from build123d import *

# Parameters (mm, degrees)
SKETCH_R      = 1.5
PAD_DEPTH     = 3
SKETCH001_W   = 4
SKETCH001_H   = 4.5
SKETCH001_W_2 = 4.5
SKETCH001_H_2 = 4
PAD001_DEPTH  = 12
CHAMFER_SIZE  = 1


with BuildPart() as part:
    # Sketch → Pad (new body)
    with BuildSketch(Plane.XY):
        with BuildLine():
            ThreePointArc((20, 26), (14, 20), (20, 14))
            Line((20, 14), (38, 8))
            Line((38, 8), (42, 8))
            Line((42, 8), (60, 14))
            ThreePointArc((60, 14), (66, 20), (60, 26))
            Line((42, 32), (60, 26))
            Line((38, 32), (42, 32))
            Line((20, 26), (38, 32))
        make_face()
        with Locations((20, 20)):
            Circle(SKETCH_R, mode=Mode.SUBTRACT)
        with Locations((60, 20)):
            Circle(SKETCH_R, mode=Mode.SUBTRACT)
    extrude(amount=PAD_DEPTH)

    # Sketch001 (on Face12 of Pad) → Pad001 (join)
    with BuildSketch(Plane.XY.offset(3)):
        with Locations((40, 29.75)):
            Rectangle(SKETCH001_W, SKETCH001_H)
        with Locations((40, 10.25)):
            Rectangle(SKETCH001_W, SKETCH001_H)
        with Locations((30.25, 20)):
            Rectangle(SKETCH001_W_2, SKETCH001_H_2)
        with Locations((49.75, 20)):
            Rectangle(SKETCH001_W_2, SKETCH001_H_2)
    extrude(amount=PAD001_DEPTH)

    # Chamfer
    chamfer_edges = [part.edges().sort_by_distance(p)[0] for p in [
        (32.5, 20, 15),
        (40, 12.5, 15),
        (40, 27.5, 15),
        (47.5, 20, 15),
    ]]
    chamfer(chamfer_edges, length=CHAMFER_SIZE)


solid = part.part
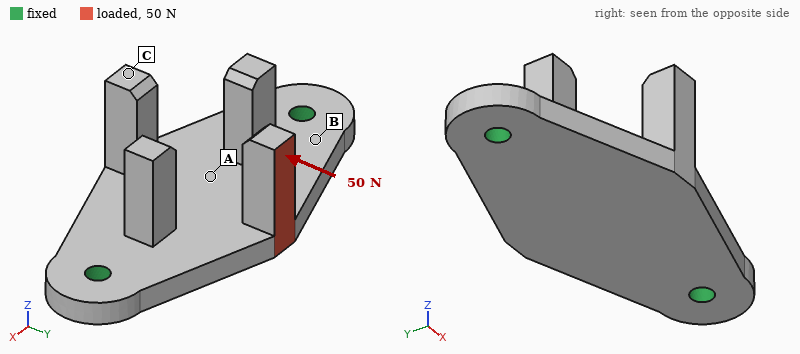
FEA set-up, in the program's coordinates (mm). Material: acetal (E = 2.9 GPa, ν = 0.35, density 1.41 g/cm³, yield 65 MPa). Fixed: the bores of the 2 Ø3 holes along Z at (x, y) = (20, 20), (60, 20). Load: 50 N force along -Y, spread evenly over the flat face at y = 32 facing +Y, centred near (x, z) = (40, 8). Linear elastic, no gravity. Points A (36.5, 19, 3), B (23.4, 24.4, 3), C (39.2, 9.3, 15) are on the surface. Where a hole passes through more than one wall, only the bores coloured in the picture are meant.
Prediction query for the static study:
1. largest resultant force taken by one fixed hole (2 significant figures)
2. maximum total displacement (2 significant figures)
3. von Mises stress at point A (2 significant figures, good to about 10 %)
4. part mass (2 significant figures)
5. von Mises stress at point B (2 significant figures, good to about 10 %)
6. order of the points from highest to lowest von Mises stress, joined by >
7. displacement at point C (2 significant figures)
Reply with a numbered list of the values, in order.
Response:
1. 25 N
2. 0.65 mm
3. 3.4 MPa
4. 4.8 g
5. 6.8 MPa
6. B > A > C
7. 0.19 mm
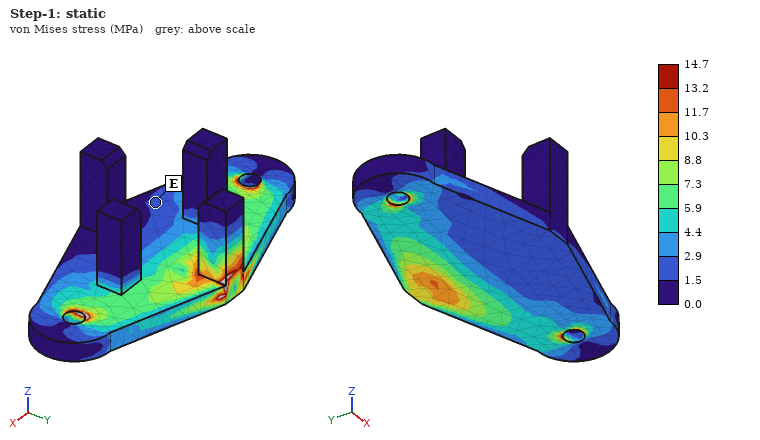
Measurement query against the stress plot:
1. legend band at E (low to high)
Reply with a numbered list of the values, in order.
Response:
1. 1.5 to 2.9 MPa
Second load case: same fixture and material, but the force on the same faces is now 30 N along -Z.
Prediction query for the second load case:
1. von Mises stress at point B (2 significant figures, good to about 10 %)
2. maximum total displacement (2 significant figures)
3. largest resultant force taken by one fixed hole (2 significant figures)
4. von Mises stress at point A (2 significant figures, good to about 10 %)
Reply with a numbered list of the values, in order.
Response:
1. 8.0 MPa
2. 0.54 mm
3. 15 N
4. 4.0 MPa
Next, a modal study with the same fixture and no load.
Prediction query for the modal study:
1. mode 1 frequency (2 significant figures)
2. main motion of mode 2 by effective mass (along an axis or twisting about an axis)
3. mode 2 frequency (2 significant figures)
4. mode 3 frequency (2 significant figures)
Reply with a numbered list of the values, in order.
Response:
1. 1600 Hz
2. along Z
3. 1800 Hz
4. 3300 Hz
